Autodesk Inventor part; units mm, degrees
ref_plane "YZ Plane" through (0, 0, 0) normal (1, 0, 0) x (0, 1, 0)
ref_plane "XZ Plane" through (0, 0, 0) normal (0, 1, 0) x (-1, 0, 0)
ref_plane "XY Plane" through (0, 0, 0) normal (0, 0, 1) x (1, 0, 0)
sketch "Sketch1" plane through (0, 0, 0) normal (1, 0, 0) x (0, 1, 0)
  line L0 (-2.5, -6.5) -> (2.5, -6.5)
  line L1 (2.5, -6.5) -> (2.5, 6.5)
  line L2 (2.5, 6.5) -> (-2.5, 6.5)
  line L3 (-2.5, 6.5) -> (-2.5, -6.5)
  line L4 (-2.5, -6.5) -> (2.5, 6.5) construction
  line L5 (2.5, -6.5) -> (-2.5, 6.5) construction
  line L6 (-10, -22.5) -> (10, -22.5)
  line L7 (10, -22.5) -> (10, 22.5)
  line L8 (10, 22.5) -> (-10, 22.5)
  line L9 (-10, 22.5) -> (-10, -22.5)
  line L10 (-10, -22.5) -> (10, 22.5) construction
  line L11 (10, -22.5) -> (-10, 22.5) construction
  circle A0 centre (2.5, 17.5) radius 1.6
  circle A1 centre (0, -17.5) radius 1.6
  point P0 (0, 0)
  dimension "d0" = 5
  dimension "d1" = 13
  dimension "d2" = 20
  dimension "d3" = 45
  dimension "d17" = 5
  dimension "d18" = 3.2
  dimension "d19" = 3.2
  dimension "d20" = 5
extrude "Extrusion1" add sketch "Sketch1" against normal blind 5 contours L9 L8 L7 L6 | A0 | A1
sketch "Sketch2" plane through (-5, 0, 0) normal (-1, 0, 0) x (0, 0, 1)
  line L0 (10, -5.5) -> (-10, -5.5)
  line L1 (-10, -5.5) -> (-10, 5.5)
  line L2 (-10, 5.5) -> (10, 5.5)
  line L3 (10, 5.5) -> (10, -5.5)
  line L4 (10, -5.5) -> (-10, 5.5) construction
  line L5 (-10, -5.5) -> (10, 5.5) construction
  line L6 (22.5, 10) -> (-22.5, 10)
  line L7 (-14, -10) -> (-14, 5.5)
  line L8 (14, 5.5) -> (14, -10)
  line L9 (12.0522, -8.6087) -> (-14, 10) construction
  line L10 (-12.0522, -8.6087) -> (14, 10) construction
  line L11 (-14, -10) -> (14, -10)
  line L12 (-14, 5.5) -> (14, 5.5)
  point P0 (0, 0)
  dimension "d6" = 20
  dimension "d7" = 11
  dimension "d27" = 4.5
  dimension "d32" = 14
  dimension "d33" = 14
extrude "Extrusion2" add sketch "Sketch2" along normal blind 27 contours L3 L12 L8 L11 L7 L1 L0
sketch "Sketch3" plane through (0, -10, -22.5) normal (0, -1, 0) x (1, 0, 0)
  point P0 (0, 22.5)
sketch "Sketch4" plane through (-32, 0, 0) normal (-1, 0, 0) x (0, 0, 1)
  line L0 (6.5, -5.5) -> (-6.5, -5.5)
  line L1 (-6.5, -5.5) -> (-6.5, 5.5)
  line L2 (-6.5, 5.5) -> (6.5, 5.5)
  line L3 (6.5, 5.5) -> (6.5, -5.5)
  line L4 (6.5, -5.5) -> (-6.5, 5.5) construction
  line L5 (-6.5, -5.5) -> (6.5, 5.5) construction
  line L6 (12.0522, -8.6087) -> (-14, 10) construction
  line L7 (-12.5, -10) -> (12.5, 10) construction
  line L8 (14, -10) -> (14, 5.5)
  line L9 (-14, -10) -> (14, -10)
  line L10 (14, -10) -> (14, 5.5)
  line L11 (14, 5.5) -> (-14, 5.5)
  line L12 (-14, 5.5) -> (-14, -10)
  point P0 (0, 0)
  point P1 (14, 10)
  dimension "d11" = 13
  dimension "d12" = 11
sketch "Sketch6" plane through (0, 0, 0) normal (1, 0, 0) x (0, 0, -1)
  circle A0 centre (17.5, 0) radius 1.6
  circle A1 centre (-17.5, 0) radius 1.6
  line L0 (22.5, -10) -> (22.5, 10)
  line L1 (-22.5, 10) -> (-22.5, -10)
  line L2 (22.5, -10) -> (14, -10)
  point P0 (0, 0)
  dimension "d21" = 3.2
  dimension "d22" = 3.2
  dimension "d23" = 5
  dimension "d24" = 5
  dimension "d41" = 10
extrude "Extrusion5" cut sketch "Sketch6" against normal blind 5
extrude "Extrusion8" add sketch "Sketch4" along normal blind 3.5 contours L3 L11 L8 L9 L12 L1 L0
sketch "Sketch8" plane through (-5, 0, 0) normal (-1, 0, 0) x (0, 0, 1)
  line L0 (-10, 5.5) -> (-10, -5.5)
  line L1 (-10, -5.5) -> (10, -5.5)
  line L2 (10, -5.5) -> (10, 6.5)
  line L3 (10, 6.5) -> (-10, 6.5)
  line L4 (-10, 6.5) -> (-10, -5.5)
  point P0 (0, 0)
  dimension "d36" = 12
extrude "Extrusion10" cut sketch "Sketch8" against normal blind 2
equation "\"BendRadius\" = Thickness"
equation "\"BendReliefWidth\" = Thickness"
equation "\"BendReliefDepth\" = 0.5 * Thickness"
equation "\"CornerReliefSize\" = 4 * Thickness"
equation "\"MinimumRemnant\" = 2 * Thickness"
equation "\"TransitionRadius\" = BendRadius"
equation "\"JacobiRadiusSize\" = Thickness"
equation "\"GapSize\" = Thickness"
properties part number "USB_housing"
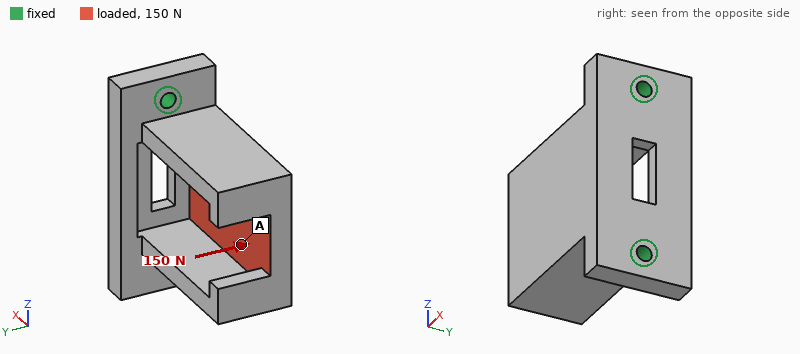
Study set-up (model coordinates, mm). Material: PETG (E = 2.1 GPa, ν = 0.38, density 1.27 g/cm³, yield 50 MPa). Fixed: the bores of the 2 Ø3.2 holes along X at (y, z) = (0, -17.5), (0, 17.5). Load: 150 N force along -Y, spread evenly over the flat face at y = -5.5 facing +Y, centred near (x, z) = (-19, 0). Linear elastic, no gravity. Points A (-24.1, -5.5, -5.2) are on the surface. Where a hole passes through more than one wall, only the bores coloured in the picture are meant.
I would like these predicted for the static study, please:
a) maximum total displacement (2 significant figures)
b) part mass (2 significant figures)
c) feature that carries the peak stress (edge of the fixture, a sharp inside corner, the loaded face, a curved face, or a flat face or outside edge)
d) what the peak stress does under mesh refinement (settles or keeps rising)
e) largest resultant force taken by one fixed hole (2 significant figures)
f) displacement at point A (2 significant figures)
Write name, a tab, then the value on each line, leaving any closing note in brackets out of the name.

maximum total displacement	0.62 mm
part mass	13 g
feature that carries the peak stress	edge of the fixture
what the peak stress does under mesh refinement	keeps rising
largest resultant force taken by one fixed hole	75 N
displacement at point A	0.40 mm
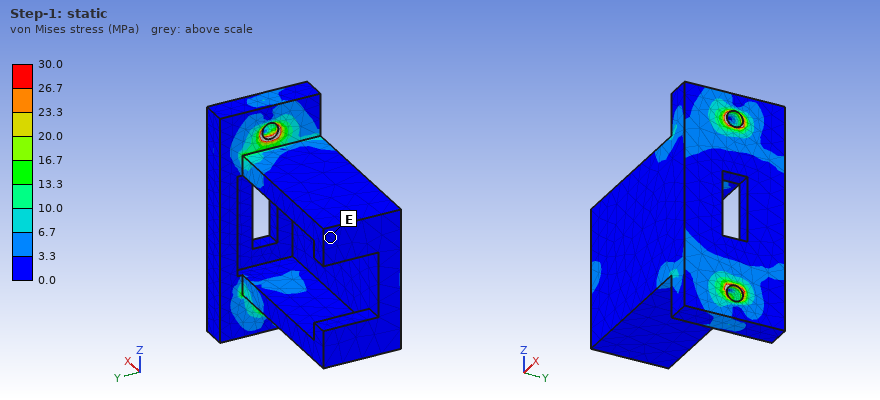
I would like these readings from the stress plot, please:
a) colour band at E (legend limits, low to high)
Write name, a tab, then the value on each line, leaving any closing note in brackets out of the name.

colour band at E	0.0 to 3.3 MPa
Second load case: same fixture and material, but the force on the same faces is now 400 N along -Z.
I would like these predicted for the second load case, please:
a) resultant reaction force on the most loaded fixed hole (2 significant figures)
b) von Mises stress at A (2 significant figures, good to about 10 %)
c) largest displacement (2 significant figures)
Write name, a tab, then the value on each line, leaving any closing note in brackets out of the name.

resultant reaction force on the most loaded fixed hole	290 N
von Mises stress at A	6.5 MPa
largest displacement	0.61 mm
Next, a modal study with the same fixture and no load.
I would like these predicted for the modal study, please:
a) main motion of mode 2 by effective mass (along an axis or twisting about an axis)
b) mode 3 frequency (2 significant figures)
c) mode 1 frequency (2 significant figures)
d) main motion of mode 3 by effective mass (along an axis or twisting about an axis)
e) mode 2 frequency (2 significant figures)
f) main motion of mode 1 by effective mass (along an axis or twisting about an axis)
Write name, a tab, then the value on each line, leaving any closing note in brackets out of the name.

main motion of mode 2 by effective mass	along Z
mode 3 frequency	3200 Hz
mode 1 frequency	950 Hz
main motion of mode 3 by effective mass	along Z
mode 2 frequency	1500 Hz
main motion of mode 1 by effective mass	along Y
